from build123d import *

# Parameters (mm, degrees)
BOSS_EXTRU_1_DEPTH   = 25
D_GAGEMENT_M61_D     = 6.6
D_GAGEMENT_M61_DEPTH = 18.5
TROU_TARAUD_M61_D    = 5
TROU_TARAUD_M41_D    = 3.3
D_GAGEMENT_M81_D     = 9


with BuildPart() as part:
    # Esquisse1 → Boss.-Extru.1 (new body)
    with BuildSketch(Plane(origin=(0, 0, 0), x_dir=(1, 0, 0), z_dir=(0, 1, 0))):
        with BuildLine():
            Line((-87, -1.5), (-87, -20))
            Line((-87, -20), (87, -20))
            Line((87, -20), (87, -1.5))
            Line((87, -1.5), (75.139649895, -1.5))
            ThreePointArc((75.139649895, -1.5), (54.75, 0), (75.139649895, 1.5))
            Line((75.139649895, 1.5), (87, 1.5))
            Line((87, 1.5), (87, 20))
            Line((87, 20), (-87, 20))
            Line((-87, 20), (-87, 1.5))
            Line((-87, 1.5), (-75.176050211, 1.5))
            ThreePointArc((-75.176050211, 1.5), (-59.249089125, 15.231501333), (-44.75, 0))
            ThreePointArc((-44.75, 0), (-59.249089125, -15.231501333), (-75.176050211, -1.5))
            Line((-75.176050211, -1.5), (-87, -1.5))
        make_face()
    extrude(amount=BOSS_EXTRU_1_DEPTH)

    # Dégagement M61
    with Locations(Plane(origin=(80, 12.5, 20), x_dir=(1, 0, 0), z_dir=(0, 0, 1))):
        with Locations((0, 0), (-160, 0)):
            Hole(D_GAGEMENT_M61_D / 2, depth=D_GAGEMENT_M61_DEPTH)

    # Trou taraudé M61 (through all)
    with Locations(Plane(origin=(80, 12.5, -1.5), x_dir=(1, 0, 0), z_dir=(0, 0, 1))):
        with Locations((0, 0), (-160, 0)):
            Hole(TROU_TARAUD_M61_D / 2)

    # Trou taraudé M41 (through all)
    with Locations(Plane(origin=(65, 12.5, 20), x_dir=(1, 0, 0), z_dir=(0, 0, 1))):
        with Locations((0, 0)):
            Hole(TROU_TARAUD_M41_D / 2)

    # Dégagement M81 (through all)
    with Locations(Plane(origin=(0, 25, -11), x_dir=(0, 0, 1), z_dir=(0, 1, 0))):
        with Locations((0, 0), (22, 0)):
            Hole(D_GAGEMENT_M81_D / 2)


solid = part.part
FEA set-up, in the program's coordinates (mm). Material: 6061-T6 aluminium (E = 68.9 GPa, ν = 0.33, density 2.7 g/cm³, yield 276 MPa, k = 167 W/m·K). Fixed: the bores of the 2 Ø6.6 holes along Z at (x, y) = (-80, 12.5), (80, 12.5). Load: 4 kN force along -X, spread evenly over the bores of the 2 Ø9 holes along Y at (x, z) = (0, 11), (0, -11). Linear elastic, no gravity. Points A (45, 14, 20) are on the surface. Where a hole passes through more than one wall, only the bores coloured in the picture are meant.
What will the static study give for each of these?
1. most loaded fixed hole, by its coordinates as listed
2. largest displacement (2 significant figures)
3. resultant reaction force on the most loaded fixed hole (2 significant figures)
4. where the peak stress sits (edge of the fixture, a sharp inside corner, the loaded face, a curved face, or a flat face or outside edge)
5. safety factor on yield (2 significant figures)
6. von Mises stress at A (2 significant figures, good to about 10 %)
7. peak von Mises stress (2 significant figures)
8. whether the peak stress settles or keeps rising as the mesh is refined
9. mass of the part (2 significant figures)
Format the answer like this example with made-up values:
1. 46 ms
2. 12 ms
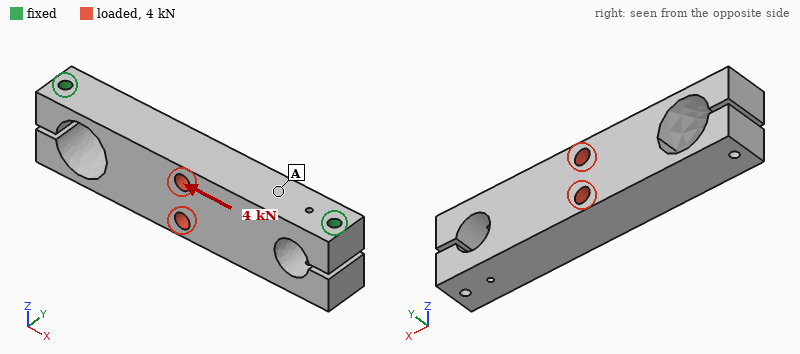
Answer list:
1. (80, 12.5)
2. 30 µm
3. 2.6 kN
4. a curved face
5. 4.4
6. 5.1 MPa
7. 63 MPa
8. settles
9. 380 g
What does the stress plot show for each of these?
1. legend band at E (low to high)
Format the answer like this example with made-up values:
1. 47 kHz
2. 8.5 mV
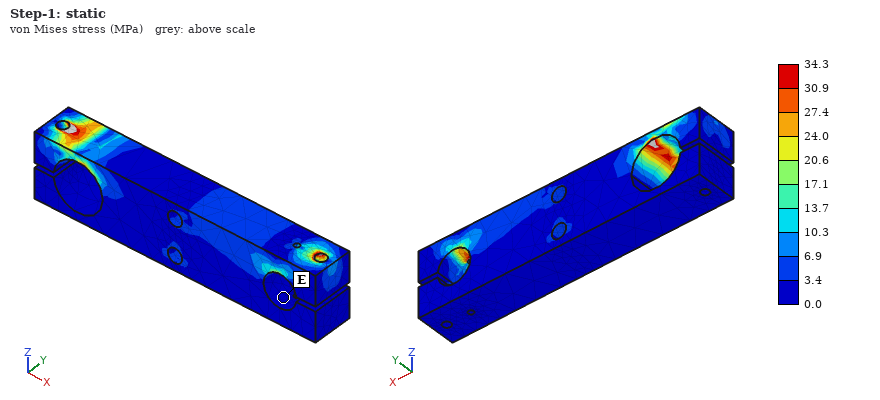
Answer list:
1. 0.0 to 3.4 MPa
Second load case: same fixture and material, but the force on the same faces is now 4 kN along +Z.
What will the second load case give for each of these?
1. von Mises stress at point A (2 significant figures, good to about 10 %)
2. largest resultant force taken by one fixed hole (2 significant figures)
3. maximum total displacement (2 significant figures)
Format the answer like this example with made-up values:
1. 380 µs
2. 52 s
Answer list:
1. 7.0 MPa
2. 2.4 kN
3. 0.11 mm
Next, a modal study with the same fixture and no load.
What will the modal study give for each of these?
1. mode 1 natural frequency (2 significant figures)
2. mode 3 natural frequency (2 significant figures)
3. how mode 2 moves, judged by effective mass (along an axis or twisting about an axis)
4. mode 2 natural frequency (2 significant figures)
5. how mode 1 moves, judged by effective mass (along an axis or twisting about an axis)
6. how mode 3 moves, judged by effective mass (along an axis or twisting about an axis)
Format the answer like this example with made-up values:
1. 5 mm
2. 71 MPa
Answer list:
1. 1200 Hz
2. 2400 Hz
3. along Z
4. 1600 Hz
5. along Y
6. along Z
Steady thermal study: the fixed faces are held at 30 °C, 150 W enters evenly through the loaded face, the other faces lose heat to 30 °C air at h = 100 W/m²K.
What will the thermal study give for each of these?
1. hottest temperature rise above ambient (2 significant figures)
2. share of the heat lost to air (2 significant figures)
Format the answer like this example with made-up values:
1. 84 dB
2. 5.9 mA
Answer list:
1. 51 K
2. 54 %
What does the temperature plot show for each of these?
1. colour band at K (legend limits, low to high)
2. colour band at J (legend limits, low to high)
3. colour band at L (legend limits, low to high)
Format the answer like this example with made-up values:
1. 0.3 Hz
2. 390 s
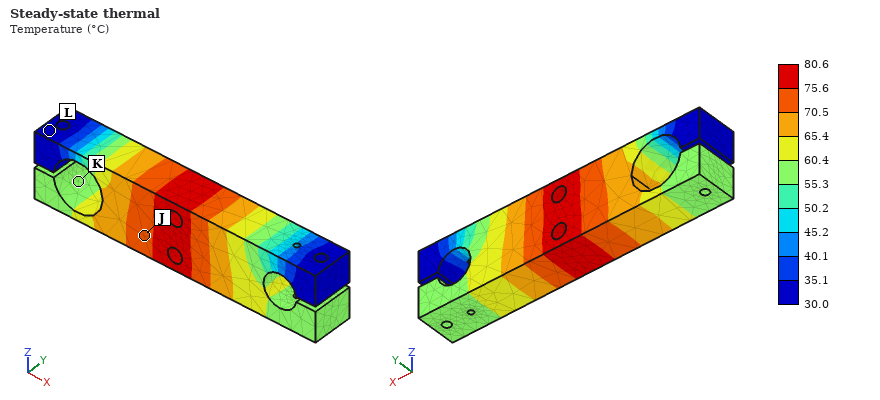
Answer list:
1. 55.3 to 60.4 °C
2. 70.5 to 75.6 °C
3. 30.0 to 35.1 °C
